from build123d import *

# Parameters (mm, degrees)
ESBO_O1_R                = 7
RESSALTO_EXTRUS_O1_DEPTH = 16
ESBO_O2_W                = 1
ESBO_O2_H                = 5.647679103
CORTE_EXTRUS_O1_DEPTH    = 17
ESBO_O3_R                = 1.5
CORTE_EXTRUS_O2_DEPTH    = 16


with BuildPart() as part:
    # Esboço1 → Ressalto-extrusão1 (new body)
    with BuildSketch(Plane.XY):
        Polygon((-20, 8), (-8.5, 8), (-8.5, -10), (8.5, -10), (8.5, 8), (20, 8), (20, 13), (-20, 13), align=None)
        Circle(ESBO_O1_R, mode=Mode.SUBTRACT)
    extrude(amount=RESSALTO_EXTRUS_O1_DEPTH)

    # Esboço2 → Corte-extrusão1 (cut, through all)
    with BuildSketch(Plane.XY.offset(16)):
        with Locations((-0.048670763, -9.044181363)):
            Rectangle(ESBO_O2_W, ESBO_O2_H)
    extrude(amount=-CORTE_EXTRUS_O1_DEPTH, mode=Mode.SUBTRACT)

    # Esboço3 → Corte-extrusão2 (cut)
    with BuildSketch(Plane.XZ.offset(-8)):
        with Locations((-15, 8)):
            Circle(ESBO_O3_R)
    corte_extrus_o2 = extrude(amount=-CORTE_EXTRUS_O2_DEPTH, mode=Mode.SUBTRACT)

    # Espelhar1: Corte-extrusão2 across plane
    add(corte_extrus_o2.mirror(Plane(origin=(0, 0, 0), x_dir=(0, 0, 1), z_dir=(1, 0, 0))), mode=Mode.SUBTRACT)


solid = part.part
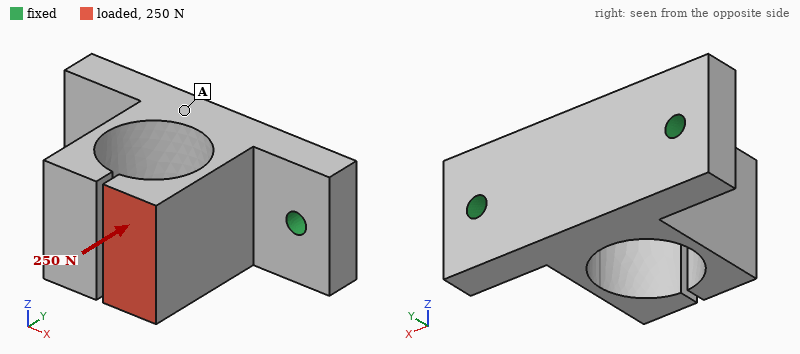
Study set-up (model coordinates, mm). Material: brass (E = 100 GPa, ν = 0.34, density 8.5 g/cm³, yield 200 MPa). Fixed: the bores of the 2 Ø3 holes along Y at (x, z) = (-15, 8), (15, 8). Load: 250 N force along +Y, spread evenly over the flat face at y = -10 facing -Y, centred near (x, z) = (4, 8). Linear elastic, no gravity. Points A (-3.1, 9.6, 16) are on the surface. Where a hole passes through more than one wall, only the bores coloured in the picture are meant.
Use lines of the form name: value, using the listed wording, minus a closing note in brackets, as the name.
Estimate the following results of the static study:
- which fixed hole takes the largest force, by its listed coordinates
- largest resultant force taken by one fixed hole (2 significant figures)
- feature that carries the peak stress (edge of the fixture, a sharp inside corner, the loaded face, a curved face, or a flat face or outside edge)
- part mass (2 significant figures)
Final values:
which fixed hole takes the largest force, by its listed coordinates: (15, 8)
largest resultant force taken by one fixed hole: 180 N
feature that carries the peak stress: a curved face
part mass: 47 g
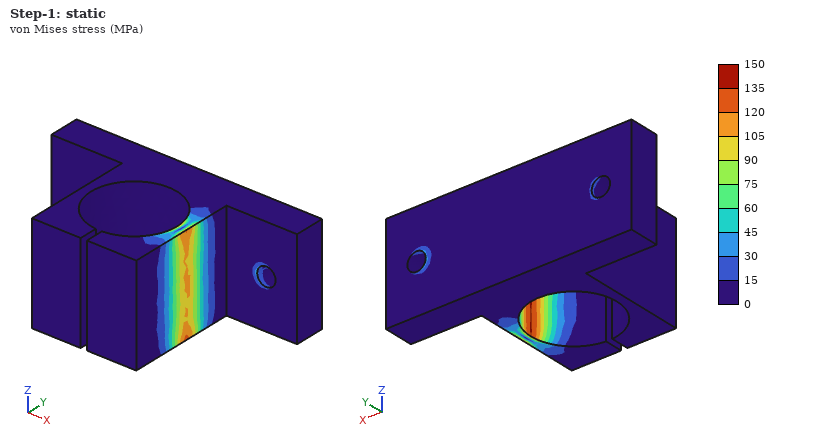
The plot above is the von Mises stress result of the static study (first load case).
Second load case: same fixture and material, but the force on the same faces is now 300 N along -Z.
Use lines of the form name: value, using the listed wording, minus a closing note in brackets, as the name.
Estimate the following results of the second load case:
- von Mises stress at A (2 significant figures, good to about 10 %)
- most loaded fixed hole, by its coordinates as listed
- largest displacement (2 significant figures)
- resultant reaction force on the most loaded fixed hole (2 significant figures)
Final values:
von Mises stress at A: 14 MPa
most loaded fixed hole, by its coordinates as listed: (15, 8)
largest displacement: 69 µm
resultant reaction force on the most loaded fixed hole: 190 N
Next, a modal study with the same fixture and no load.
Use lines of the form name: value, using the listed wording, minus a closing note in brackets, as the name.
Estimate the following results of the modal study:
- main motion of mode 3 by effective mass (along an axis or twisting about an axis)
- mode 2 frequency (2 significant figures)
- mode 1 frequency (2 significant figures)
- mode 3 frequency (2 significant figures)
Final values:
main motion of mode 3 by effective mass: along Z
mode 2 frequency: 2300 Hz
mode 1 frequency: 2300 Hz
mode 3 frequency: 4700 Hz
